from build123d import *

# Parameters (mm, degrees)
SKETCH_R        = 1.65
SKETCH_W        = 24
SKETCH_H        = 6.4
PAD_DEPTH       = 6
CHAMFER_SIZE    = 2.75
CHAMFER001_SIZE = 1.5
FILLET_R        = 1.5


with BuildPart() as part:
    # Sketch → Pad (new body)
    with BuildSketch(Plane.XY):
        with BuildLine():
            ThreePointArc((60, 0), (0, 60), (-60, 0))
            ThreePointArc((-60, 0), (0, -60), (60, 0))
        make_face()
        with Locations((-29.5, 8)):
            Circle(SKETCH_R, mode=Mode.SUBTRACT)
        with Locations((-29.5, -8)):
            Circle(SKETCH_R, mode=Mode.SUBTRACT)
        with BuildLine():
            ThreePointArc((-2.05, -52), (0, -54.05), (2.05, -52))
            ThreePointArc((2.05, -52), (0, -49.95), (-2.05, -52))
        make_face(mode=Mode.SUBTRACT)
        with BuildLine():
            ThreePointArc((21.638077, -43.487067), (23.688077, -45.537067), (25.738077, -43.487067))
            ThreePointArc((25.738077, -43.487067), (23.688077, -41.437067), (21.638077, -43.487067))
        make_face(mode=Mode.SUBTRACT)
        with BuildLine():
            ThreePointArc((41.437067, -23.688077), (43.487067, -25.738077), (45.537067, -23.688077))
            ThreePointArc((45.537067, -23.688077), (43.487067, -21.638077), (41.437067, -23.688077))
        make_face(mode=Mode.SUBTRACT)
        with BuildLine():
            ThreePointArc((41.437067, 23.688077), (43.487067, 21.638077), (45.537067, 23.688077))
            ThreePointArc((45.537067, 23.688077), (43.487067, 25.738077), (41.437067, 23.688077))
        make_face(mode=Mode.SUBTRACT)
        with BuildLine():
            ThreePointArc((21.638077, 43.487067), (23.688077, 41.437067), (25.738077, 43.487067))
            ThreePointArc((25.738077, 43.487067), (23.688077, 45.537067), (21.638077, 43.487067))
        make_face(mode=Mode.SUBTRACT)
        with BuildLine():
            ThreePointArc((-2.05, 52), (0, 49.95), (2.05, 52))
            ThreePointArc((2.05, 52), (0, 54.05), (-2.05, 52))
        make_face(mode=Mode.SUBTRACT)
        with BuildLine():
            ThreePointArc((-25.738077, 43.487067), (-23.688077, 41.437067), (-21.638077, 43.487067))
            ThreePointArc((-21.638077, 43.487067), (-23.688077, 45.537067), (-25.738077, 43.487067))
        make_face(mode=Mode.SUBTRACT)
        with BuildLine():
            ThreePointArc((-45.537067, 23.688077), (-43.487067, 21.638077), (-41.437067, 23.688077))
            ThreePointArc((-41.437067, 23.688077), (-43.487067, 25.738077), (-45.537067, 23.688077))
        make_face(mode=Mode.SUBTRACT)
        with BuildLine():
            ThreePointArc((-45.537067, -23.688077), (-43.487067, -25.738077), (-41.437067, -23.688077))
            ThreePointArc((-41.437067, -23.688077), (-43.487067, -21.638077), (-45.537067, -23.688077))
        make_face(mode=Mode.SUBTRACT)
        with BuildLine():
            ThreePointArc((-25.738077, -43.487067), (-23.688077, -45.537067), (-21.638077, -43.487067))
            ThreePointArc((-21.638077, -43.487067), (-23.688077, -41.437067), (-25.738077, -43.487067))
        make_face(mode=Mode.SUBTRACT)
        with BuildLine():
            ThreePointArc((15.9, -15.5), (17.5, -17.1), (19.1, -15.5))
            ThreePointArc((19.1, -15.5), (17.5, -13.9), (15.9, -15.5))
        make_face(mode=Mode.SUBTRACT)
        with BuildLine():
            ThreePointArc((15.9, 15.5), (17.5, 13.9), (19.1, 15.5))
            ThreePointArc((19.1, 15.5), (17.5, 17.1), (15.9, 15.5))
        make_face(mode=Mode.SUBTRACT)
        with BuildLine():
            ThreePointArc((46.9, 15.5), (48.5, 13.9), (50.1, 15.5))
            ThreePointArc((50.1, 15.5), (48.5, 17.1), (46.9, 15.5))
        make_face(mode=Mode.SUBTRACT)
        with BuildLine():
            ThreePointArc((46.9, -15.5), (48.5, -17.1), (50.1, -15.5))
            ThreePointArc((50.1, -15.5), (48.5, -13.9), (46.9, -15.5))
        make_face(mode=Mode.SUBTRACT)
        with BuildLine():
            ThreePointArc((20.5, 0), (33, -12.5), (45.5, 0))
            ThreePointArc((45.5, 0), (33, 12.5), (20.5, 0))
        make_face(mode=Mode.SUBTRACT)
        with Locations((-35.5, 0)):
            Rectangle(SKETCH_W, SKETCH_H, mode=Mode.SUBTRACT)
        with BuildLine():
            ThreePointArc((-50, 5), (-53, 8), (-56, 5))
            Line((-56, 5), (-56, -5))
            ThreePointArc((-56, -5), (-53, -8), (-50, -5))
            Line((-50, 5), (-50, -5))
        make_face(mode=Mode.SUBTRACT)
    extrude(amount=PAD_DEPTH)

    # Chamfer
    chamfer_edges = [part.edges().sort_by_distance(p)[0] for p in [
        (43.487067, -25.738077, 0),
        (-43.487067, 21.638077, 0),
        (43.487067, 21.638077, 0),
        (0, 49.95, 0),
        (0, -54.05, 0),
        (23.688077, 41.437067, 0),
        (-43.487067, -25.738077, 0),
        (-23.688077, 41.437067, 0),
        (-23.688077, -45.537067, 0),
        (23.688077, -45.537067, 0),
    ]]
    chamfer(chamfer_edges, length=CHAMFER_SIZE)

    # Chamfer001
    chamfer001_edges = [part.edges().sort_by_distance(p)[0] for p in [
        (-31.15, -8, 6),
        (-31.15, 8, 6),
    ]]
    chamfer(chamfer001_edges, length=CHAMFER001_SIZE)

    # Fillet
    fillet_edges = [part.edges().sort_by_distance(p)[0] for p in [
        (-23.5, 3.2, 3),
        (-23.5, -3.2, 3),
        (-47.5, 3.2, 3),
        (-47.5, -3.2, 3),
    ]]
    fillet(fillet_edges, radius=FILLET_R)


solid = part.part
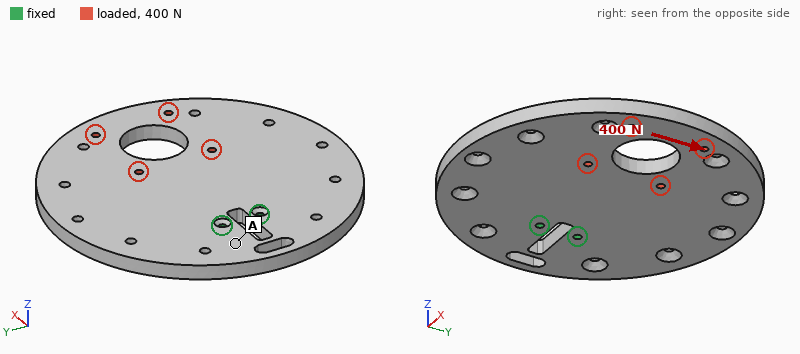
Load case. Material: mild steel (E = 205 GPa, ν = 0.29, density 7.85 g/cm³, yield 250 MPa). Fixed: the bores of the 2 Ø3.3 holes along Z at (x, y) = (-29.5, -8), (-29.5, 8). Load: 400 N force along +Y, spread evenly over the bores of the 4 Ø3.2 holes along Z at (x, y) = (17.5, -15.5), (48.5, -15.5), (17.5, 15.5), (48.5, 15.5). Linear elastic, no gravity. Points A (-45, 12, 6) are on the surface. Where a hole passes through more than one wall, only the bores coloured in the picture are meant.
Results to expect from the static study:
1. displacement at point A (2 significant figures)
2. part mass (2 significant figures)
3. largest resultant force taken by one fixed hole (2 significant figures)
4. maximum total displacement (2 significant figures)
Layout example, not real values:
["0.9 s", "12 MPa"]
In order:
["3.1 µm", "480 g", "1.2 kN", "16 µm"]
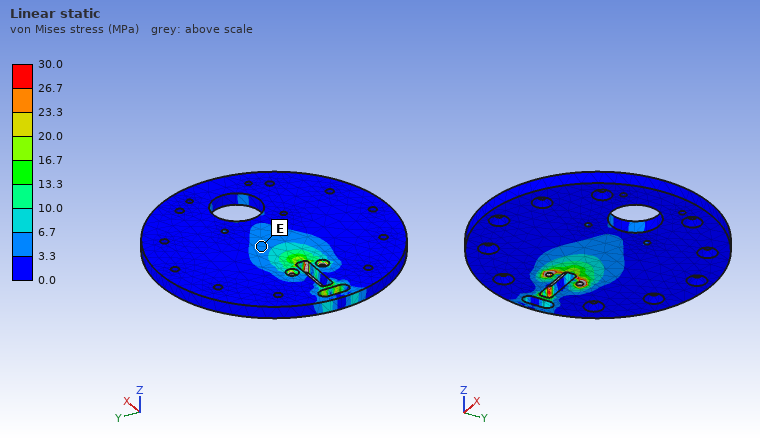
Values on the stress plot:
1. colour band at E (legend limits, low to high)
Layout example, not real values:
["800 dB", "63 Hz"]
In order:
["3.3 to 6.7 MPa"]
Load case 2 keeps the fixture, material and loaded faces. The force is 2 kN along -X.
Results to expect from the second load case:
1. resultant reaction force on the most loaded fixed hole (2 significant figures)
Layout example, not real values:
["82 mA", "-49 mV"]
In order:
["1.0 kN"]
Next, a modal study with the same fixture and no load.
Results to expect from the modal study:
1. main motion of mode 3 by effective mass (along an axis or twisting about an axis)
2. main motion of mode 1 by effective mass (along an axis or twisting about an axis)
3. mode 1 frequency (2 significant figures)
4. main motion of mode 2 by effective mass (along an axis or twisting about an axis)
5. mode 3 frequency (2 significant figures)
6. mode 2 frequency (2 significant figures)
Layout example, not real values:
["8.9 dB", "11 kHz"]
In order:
["along Y", "along Z", "560 Hz", "twisting about X", "1700 Hz", "980 Hz"]
